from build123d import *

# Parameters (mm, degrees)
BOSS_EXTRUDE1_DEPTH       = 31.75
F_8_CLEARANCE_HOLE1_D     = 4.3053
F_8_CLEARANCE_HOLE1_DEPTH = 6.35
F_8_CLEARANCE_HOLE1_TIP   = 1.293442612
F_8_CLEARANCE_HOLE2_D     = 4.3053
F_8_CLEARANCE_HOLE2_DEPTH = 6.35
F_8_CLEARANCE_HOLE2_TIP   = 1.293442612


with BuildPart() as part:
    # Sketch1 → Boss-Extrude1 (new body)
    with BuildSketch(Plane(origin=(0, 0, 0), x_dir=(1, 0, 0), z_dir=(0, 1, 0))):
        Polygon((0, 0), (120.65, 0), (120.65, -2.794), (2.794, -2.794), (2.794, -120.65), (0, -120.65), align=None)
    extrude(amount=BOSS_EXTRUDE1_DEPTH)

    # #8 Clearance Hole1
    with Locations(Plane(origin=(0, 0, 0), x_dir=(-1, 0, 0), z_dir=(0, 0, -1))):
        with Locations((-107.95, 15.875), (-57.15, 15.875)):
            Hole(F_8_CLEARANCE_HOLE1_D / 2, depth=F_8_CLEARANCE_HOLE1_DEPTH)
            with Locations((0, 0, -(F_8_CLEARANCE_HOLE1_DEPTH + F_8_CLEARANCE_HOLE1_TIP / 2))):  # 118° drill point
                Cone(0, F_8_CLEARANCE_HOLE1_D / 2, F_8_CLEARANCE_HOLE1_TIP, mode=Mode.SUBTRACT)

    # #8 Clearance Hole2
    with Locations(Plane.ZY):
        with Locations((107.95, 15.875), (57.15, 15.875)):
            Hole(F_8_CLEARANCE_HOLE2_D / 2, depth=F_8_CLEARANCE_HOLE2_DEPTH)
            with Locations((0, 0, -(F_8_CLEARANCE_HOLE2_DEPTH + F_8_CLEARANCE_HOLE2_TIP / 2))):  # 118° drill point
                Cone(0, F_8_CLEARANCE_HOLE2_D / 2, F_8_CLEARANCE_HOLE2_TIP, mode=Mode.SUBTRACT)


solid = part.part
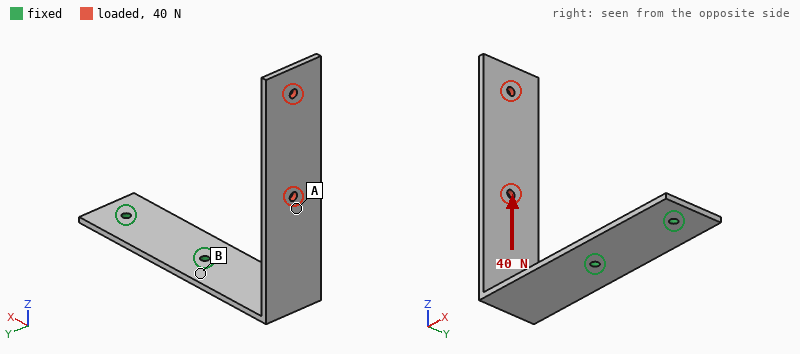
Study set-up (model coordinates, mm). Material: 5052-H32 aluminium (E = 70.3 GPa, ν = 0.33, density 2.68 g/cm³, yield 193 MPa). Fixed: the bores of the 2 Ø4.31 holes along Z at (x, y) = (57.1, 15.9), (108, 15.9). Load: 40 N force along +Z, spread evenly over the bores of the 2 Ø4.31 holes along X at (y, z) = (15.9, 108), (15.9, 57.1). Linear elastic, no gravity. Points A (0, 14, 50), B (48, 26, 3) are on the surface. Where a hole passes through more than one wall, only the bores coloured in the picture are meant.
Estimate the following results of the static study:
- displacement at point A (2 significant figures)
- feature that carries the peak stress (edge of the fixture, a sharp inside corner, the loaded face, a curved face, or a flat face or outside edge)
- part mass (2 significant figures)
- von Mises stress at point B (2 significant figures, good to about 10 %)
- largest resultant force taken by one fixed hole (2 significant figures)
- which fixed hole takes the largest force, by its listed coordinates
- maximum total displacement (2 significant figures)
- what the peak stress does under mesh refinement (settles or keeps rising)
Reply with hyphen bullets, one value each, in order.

- 0.95 mm
- edge of the fixture
- 56 g
- 42 MPa
- 47 N
- (57.1, 15.9)
- 1.9 mm
- keeps rising
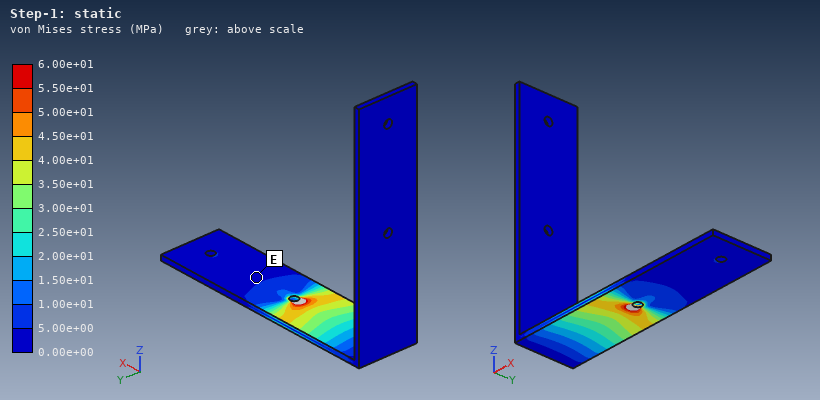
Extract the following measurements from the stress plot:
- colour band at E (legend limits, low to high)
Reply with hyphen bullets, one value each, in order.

- 0.00e+00 to 5.00e+00 MPa
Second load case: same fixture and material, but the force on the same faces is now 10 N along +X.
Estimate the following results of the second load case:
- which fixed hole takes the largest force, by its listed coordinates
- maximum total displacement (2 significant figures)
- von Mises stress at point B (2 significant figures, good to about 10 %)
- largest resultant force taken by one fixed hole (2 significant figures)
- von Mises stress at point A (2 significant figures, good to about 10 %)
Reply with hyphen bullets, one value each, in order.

- (57.1, 15.9)
- 2.1 mm
- 19 MPa
- 8.8 N
- 7.5 MPa
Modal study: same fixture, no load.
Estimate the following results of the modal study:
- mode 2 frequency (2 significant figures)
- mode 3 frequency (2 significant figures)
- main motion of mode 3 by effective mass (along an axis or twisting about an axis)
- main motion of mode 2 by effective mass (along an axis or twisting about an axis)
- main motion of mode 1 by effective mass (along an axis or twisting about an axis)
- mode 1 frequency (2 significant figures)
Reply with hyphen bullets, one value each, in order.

- 140 Hz
- 340 Hz
- along Z
- along Y
- along X
- 94 Hz
